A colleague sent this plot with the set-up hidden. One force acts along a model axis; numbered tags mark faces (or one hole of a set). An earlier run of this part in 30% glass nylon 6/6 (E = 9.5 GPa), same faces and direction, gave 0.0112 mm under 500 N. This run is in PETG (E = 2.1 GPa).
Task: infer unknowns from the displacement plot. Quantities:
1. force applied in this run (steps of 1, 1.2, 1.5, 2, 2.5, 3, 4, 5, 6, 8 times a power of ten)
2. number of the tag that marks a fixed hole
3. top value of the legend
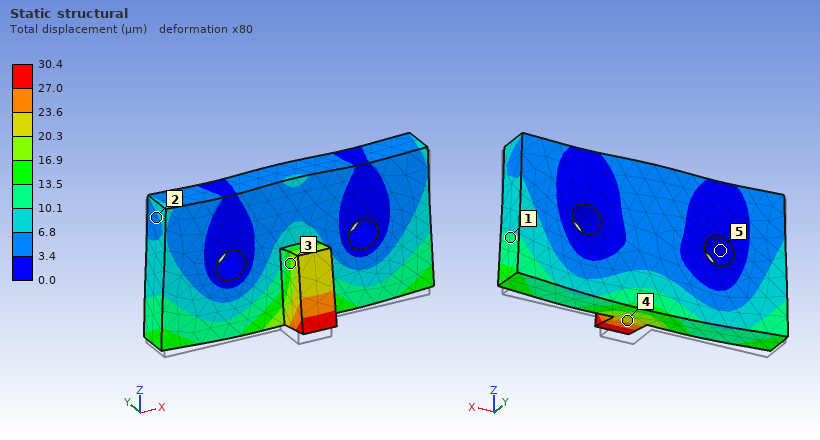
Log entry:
300 N
5
30.4 µm
